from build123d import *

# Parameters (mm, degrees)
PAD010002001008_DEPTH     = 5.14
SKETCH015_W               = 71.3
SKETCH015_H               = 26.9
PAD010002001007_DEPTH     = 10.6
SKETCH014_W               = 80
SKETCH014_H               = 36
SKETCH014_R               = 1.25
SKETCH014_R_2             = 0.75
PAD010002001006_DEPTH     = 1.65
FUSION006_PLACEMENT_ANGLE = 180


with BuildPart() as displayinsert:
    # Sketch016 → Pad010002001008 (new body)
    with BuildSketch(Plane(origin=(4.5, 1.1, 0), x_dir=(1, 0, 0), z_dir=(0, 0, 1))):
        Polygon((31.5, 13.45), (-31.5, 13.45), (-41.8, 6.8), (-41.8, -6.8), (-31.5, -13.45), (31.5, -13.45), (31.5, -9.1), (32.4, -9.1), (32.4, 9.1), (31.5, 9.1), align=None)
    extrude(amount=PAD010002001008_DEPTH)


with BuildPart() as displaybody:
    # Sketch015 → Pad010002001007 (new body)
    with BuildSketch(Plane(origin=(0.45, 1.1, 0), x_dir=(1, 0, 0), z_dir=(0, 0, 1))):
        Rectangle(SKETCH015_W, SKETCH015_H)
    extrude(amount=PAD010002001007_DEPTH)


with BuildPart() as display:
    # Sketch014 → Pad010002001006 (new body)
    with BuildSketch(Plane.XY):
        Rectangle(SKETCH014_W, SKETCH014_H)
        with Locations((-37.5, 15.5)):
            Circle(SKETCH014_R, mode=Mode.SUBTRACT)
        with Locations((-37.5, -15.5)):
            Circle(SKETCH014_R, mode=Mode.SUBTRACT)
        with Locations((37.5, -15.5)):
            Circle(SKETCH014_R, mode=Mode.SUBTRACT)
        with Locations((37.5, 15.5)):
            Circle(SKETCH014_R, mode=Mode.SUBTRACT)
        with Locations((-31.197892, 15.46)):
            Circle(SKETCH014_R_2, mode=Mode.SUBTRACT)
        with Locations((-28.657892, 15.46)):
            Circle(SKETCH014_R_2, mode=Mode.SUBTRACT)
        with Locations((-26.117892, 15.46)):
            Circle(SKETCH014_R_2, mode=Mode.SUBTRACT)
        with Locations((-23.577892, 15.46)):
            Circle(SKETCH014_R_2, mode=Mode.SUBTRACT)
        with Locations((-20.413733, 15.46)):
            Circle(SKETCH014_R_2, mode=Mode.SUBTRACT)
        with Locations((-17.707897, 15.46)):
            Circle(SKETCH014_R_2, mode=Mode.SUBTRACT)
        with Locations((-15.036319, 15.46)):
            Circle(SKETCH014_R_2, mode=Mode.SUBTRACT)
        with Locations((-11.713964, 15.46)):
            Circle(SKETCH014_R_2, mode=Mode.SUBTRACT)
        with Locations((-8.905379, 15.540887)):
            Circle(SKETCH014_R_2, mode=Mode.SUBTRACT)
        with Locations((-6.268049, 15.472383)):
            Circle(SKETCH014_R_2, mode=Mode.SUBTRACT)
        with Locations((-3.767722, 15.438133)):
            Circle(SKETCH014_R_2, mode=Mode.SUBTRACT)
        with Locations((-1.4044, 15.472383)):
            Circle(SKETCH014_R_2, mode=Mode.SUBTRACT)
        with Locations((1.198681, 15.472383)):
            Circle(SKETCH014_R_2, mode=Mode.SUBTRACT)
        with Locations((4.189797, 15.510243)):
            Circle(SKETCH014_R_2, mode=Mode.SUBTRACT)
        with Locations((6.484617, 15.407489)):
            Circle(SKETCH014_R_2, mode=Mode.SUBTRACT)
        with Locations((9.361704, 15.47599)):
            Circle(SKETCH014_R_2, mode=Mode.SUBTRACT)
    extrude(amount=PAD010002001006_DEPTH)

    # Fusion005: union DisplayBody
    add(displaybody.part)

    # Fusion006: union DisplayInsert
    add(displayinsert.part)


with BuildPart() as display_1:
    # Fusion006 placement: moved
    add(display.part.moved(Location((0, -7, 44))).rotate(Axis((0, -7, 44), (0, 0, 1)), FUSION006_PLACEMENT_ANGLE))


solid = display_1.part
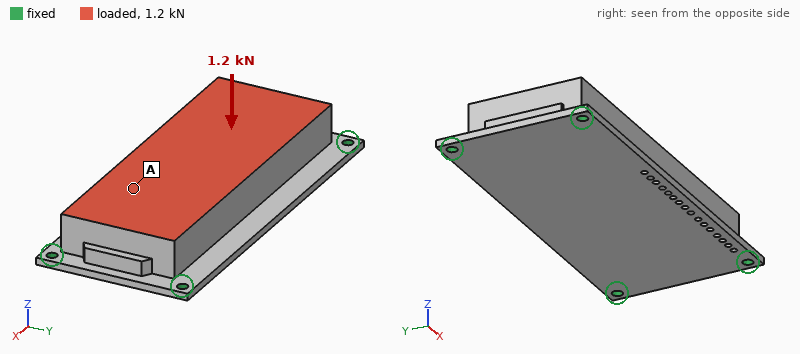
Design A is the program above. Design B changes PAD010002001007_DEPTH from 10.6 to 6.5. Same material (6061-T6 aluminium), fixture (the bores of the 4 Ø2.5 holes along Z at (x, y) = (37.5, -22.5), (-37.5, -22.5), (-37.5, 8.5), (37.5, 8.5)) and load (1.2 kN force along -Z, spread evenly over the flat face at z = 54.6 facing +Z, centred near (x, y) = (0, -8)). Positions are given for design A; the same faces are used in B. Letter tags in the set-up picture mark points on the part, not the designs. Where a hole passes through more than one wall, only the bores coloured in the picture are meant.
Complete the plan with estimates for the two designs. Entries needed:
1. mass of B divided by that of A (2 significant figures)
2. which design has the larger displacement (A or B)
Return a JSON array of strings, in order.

["0.64", "B"]
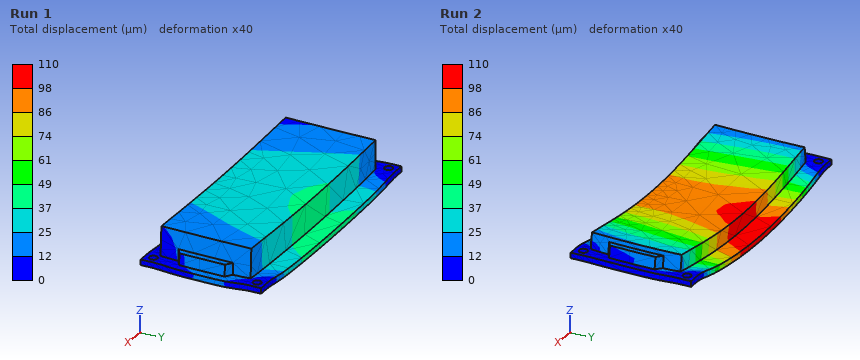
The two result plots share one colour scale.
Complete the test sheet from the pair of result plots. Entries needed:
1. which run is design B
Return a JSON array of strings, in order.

["Run 2"]
